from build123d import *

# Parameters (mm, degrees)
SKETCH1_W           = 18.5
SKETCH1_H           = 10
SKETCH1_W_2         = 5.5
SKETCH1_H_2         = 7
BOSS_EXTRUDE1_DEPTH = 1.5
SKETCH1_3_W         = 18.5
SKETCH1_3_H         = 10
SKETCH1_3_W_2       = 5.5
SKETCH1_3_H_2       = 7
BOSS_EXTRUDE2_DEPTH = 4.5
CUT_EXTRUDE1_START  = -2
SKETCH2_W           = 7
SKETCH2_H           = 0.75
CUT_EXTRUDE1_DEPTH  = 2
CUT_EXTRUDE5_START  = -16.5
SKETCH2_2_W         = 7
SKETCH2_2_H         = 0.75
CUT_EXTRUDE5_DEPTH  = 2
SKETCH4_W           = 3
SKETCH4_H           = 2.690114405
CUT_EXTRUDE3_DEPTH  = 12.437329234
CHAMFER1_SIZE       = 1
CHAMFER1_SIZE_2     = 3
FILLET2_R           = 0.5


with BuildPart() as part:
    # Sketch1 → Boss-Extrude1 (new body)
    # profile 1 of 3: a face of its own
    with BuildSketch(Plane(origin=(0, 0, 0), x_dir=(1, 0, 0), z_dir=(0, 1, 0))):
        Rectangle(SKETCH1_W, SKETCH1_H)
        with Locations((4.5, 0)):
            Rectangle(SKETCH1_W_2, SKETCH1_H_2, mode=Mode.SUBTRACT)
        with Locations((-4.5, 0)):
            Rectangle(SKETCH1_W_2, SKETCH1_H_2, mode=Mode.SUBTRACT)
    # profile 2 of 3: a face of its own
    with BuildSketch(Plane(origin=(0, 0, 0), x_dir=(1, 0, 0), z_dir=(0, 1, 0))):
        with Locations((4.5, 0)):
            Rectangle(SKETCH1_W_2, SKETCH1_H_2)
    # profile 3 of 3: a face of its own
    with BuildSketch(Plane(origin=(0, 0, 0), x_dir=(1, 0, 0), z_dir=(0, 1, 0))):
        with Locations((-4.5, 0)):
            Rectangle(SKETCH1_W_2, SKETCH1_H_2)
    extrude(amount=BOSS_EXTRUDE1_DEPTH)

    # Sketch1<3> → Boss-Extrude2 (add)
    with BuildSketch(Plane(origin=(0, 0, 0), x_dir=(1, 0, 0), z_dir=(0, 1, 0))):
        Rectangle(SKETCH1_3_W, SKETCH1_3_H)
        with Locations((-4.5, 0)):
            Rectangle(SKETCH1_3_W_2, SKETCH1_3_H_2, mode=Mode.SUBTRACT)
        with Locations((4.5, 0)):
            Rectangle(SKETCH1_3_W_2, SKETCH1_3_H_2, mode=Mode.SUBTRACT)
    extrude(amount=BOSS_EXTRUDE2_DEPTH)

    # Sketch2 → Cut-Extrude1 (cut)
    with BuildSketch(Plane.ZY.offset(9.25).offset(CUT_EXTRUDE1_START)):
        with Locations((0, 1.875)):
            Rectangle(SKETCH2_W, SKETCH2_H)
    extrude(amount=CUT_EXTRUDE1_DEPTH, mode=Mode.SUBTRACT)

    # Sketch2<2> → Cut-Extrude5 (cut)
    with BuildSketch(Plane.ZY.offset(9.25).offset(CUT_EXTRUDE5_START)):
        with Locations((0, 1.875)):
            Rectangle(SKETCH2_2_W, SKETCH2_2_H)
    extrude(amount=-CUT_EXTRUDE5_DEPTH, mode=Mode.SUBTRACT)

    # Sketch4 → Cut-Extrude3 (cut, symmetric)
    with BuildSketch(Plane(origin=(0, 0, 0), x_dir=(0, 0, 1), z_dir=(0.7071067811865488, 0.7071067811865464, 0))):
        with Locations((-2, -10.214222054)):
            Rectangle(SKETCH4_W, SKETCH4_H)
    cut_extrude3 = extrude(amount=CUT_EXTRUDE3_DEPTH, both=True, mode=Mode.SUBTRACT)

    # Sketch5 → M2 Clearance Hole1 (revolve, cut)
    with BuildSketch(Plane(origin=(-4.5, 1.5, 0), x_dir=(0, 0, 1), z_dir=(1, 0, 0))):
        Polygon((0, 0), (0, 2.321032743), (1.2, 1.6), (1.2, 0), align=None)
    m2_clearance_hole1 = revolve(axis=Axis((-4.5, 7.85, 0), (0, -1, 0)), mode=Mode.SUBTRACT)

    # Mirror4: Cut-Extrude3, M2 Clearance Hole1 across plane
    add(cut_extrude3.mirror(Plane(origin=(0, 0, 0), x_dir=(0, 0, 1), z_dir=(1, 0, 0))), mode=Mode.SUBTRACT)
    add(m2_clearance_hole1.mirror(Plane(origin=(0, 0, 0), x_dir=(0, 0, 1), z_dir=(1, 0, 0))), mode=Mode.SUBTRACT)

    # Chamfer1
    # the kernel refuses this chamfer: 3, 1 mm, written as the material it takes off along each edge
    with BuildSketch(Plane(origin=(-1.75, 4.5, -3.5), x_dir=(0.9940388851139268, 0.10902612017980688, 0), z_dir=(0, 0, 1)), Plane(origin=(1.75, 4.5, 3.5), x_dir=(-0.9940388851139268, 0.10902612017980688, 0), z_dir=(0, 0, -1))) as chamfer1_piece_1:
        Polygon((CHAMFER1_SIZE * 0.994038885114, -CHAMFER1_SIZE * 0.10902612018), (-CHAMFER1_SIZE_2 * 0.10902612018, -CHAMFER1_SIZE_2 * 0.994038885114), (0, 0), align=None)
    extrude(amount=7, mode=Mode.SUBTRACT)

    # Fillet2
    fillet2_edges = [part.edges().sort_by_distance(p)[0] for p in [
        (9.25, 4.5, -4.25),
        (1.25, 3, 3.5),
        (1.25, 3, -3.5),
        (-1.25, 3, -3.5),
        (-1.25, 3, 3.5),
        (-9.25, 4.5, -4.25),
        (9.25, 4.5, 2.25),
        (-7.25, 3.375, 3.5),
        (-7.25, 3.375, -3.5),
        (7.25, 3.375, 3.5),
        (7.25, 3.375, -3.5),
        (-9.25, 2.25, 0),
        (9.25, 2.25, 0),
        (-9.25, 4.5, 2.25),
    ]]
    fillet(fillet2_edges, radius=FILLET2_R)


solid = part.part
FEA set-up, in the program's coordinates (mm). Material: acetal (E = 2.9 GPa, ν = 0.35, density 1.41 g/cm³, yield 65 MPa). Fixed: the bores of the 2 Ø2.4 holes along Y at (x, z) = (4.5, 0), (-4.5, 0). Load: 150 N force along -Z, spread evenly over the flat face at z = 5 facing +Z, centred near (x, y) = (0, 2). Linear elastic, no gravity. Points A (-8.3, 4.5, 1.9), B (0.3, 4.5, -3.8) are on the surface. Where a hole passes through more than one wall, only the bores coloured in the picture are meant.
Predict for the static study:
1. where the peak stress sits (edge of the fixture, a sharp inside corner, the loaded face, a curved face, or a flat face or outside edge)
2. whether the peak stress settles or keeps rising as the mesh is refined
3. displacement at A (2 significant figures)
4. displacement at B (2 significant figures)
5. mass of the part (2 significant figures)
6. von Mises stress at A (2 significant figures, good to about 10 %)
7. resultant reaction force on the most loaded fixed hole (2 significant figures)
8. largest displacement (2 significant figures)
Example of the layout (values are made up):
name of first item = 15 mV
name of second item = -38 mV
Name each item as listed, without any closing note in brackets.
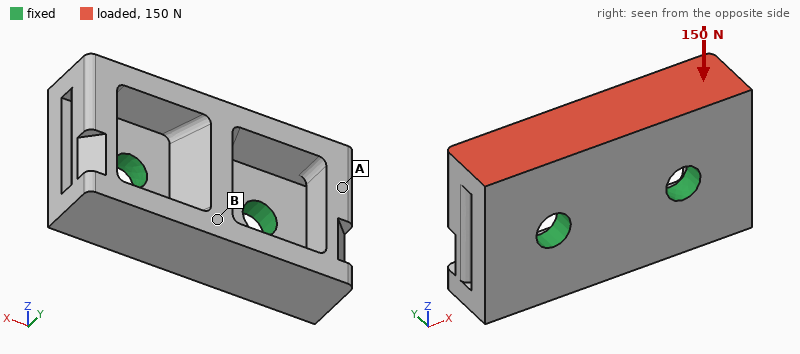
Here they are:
where the peak stress sits = edge of the fixture
whether the peak stress settles or keeps rising as the mesh is refined = keeps rising
displacement at A = 0.069 mm
displacement at B = 0.055 mm
mass of the part = 0.76 g
von Mises stress at A = 6.5 MPa
resultant reaction force on the most loaded fixed hole = 75 N
largest displacement = 0.11 mm
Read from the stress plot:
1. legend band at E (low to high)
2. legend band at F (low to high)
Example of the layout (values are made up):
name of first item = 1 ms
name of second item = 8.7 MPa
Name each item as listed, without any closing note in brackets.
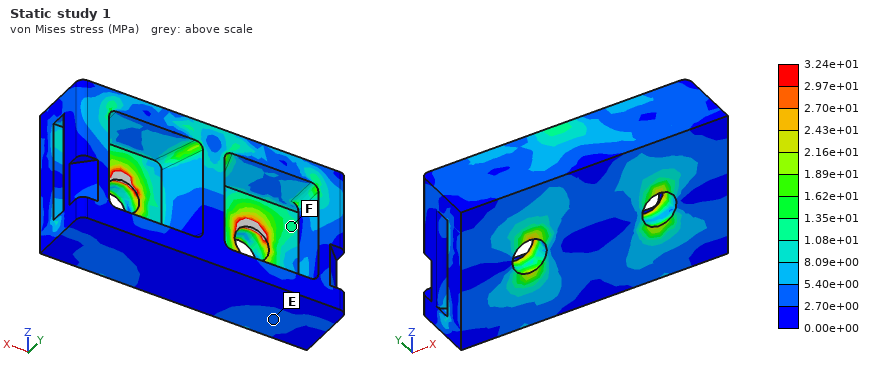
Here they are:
legend band at E = 2.70e+00 to 5.40e+00 MPa
legend band at F = 1.08e+01 to 1.35e+01 MPa
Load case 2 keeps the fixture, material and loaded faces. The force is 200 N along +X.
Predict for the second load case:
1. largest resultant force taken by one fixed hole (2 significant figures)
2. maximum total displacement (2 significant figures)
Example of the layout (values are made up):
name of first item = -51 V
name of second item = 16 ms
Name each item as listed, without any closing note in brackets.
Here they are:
largest resultant force taken by one fixed hole = 140 N
maximum total displacement = 87 µm
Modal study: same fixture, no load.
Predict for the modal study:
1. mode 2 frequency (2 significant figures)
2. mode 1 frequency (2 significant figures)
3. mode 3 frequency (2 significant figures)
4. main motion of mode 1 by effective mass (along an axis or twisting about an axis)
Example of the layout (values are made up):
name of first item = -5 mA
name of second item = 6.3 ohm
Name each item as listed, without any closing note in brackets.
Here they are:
mode 2 frequency = 9900 Hz
mode 1 frequency = 7600 Hz
mode 3 frequency = 11 kHz
main motion of mode 1 by effective mass = along Z
